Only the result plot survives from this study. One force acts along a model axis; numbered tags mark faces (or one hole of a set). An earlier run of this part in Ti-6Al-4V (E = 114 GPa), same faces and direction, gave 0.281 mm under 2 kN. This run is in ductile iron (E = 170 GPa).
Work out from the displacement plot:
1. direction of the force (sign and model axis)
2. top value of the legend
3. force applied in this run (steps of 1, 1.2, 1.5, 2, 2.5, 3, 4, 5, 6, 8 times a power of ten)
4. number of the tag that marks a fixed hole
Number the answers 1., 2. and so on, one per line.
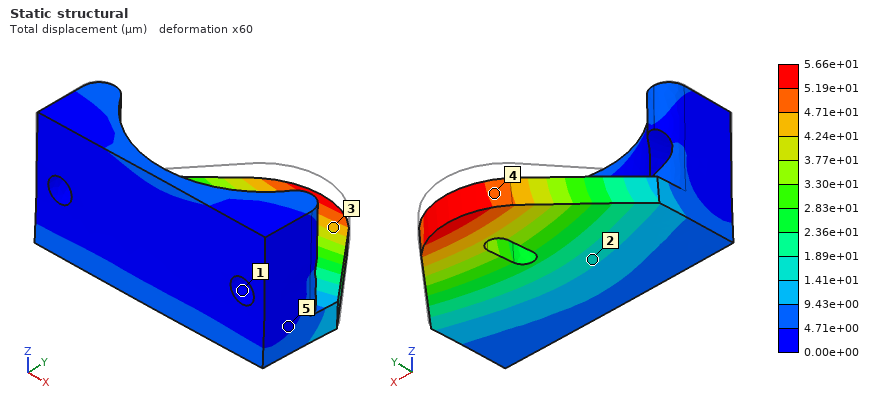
1. -Z
2. 5.66e+01 µm
3. 600 N
4. 1
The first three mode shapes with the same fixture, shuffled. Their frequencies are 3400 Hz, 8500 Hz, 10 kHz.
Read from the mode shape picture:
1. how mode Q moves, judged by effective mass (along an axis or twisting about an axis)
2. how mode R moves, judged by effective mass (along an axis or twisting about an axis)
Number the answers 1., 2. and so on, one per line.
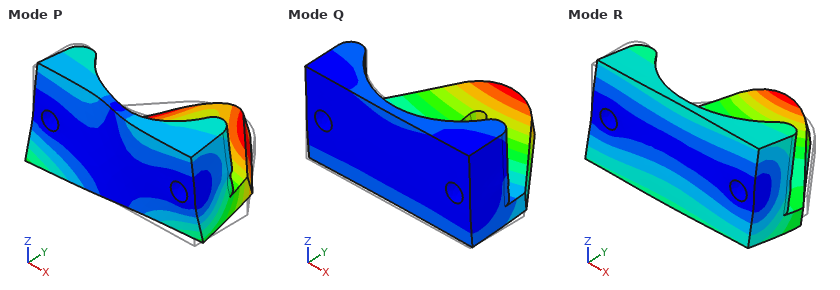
1. along Z
2. along Y
